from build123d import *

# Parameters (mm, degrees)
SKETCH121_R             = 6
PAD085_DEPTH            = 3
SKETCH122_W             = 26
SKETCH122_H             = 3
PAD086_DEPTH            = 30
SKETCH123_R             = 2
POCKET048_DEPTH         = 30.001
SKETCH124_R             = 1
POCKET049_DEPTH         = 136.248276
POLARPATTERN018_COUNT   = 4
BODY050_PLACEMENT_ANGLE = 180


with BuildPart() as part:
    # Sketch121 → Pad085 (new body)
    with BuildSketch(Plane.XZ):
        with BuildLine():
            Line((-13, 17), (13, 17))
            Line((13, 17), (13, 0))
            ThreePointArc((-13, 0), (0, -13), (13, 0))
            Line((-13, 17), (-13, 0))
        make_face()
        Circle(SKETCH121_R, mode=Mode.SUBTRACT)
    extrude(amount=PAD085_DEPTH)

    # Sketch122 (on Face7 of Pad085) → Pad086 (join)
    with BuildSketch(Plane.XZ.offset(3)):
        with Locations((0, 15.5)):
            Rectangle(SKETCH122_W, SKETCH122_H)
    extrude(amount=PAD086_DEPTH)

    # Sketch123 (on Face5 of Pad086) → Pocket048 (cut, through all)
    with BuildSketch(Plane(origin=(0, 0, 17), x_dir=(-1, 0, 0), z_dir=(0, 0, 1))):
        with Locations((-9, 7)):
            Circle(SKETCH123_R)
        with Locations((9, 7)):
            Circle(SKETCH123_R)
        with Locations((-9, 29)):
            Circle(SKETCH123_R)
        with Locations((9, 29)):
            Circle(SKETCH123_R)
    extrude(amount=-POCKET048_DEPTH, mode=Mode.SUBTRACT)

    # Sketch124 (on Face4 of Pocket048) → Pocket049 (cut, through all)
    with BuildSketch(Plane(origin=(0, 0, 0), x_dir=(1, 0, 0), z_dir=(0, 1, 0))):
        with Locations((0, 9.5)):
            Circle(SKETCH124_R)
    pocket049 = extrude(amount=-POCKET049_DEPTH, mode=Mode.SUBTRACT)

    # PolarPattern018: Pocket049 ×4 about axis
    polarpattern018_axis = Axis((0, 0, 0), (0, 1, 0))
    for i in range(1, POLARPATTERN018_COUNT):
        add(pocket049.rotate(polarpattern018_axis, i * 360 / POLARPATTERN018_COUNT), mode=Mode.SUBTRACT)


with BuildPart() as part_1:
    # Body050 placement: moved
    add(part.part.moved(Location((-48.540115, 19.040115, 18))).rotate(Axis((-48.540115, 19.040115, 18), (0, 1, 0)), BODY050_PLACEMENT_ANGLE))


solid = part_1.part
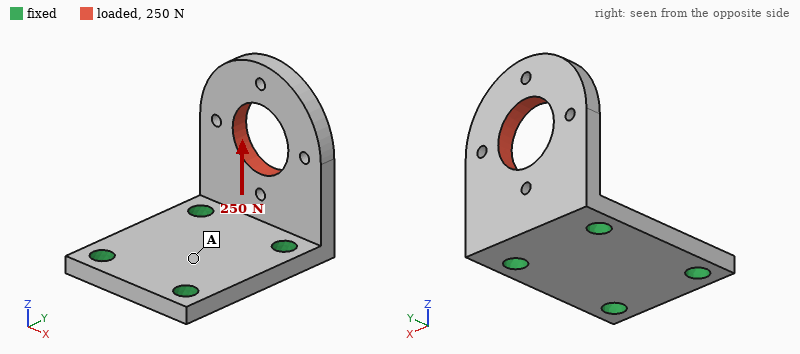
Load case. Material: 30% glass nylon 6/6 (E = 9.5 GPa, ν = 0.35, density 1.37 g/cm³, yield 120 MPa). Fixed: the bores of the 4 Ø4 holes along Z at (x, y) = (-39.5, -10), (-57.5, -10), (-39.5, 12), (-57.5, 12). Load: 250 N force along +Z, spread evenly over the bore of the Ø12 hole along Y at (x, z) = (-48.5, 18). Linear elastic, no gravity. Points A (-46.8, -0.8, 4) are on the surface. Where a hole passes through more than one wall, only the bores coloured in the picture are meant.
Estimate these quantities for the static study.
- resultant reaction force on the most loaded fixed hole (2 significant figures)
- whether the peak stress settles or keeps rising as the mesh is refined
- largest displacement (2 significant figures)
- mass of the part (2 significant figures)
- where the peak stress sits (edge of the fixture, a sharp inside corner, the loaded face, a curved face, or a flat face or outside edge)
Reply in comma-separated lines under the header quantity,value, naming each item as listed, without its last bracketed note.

quantity,value
resultant reaction force on the most loaded fixed hole,130 N
whether the peak stress settles or keeps rising as the mesh is refined,keeps rising
largest displacement,0.15 mm
mass of the part,5.4 g
where the peak stress sits,edge of the fixture
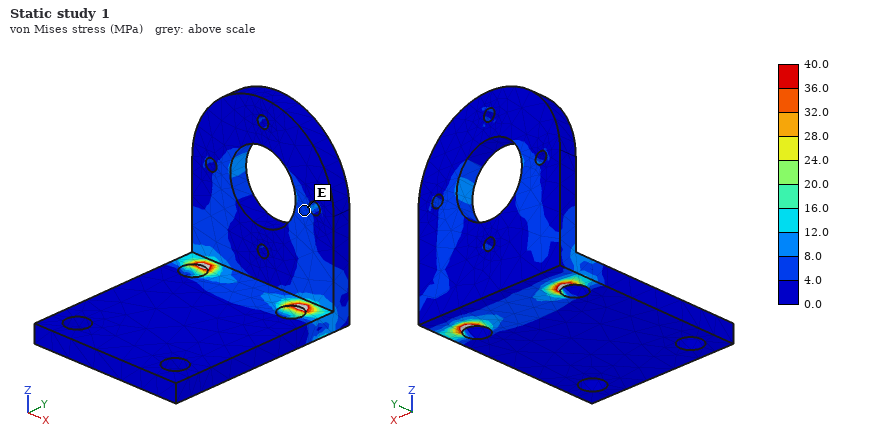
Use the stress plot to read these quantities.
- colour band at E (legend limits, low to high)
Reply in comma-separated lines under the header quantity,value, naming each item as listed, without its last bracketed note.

quantity,value
colour band at E,4.0 to 8.0 MPa
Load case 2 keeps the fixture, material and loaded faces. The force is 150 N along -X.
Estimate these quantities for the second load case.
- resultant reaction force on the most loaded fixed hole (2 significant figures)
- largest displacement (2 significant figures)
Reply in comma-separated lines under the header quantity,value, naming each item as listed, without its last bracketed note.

quantity,value
resultant reaction force on the most loaded fixed hole,140 N
largest displacement,86 µm
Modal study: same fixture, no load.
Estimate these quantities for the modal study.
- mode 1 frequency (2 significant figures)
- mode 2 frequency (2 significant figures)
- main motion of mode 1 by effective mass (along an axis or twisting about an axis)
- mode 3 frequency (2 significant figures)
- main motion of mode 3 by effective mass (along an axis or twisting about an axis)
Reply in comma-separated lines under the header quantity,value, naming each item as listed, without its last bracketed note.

quantity,value
mode 1 frequency,1600 Hz
mode 2 frequency,4100 Hz
main motion of mode 1 by effective mass,along Y
mode 3 frequency,6200 Hz
main motion of mode 3 by effective mass,along X
